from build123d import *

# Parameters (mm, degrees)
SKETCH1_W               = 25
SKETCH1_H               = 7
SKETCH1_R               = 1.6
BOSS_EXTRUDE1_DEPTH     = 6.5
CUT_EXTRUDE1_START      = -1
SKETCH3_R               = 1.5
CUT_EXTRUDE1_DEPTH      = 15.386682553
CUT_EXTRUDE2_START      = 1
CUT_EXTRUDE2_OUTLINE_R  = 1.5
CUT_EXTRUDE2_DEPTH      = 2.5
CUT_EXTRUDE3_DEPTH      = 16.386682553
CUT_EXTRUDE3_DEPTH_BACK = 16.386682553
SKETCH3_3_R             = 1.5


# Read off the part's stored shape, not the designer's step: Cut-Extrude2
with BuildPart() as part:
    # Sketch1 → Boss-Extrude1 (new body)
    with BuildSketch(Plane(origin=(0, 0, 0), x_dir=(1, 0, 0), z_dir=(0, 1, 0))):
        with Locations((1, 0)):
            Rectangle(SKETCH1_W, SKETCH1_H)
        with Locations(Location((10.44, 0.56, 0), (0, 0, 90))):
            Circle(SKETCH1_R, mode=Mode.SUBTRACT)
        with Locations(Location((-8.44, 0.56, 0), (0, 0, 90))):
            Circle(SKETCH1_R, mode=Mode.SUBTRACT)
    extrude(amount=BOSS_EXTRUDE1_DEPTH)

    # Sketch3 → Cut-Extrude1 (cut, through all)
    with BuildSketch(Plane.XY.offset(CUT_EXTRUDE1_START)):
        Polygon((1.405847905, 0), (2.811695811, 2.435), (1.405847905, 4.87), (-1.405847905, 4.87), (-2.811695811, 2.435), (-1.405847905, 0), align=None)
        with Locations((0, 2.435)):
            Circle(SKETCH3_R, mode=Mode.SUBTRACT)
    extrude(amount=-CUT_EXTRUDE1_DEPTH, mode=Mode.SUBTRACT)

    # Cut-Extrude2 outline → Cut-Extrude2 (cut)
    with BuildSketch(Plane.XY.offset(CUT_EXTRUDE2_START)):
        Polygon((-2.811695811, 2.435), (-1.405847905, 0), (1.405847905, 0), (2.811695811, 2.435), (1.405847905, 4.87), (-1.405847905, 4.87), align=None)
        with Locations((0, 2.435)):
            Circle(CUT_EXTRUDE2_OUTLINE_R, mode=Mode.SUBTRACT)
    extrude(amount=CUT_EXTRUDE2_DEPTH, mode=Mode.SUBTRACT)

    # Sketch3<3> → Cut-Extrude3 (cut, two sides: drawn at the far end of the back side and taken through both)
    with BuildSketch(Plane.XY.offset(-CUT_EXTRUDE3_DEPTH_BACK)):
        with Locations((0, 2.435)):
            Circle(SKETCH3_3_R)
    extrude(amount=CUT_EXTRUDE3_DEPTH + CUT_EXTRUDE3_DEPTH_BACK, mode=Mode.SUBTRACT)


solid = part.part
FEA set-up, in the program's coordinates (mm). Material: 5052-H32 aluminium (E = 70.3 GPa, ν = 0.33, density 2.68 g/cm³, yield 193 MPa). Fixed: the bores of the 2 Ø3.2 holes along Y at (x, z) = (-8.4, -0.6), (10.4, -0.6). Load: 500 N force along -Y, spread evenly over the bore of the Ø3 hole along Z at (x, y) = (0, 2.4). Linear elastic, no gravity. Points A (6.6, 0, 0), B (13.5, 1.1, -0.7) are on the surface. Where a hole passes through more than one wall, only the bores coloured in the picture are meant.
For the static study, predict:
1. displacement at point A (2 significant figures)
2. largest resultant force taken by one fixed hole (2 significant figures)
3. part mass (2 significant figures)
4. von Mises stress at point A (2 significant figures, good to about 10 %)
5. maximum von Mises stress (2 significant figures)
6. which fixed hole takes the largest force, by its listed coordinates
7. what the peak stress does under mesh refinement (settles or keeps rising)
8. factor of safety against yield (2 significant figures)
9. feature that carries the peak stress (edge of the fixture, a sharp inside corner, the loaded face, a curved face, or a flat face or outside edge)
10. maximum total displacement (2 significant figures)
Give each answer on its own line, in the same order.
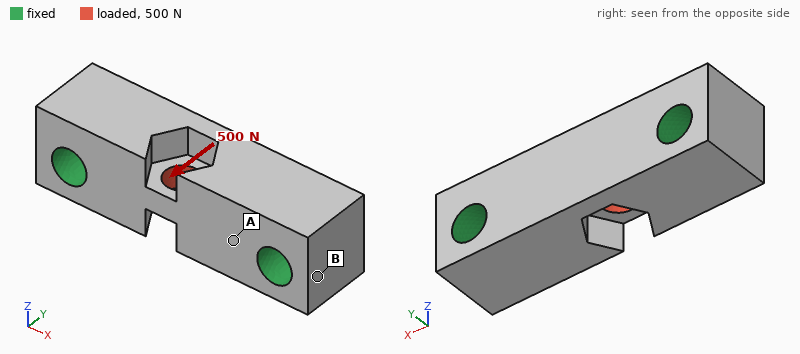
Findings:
1.4 µm
280 N
2.5 g
16 MPa
100 MPa
(-8.4, -0.6)
settles
1.9
a flat face or outside edge
6.6 µm
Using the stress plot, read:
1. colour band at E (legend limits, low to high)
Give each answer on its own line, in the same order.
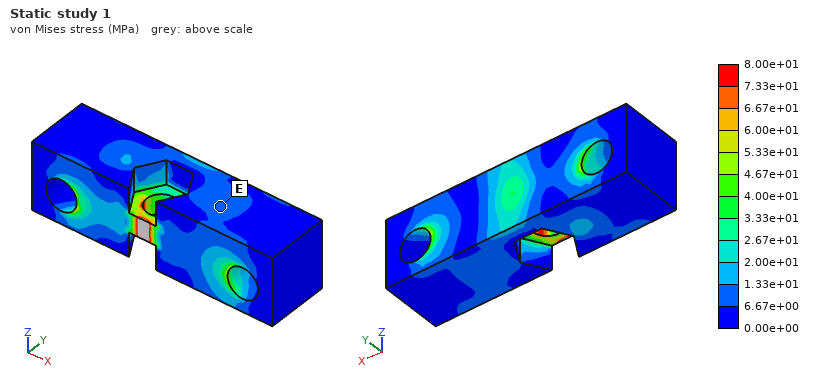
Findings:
6.67e+00 to 1.33e+01 MPa
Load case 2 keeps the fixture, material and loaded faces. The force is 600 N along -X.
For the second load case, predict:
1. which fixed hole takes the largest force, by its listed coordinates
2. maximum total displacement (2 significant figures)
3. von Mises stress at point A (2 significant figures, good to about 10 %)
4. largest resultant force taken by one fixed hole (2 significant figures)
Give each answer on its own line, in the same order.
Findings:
(-8.4, -0.6)
2.2 µm
13 MPa
320 N
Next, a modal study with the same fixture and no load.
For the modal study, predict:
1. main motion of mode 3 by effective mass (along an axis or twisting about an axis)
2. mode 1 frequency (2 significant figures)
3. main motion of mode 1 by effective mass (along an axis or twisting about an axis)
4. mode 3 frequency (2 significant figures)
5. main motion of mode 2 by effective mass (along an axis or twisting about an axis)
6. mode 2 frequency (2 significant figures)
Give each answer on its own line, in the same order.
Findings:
twisting about X
63 kHz
along Z
91 kHz
along Y
73 kHz
